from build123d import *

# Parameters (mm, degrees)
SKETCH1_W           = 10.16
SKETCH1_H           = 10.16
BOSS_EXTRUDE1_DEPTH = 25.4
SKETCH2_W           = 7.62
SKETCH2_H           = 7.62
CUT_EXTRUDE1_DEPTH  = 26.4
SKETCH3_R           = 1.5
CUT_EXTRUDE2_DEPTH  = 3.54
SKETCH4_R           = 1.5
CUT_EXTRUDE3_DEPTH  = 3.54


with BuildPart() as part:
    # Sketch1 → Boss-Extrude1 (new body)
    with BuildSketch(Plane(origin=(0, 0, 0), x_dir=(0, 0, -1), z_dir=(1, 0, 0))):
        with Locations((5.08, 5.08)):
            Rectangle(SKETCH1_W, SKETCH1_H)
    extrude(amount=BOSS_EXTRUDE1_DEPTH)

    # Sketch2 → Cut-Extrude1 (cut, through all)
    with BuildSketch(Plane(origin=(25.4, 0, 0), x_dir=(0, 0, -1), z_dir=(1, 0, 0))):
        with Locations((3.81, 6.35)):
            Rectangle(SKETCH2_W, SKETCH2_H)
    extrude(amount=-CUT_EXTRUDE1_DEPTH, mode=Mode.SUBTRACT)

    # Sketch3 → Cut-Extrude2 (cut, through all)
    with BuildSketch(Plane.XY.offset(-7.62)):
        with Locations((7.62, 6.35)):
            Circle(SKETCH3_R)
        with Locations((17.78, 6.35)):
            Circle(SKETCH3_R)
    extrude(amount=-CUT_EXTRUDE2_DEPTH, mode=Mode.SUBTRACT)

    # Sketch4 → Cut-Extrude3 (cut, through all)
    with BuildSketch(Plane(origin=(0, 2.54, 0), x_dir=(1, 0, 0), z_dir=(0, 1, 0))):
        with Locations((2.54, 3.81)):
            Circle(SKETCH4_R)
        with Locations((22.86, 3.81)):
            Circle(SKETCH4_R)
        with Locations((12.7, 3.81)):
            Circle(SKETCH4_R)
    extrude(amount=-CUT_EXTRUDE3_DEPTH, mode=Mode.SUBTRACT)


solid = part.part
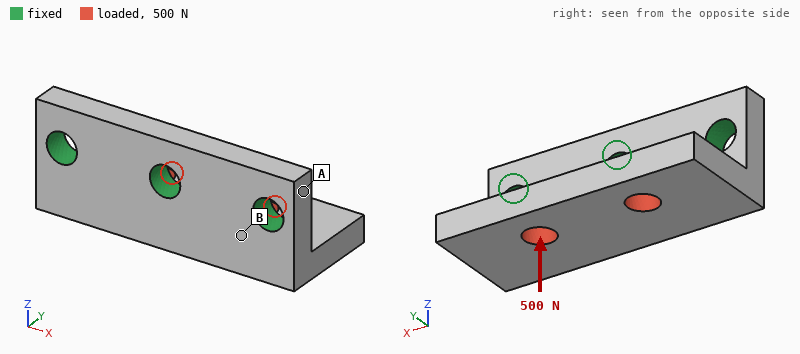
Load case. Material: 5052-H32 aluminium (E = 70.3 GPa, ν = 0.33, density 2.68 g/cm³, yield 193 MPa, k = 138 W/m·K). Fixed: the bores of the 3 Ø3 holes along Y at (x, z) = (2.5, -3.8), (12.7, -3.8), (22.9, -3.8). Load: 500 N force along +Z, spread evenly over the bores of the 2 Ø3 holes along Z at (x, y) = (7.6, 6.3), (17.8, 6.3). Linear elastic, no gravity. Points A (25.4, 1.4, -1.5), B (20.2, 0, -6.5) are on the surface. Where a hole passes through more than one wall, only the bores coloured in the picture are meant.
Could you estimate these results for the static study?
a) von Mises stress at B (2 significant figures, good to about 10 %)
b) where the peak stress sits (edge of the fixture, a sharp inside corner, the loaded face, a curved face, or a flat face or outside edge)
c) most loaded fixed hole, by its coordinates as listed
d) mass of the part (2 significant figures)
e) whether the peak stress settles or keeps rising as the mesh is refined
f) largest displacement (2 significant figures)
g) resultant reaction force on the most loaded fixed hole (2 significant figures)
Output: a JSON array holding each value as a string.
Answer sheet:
["63 MPa", "edge of the fixture", "(12.7, -3.8)", "2.8 g", "keeps rising", "58 µm", "300 N"]
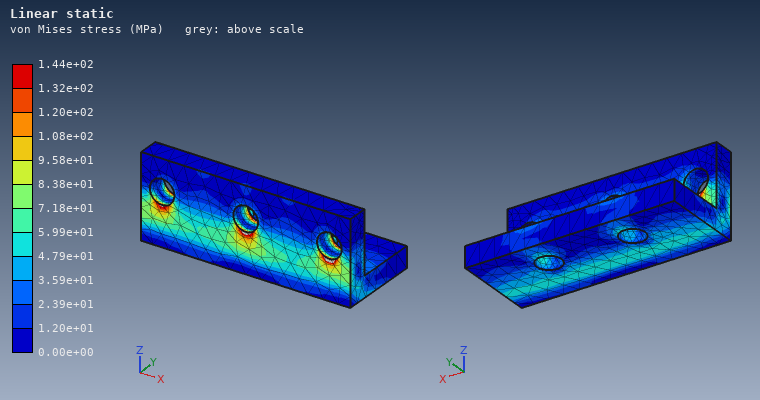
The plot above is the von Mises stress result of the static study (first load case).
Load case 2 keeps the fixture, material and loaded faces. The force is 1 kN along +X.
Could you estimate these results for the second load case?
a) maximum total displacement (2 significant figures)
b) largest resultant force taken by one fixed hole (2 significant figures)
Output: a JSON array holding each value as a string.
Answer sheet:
["22 µm", "440 N"]
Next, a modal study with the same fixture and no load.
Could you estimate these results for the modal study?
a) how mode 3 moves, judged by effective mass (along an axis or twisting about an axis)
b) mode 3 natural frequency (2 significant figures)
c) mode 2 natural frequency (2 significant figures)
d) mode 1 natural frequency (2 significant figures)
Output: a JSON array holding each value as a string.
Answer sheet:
["along X", "41 kHz", "22 kHz", "16 kHz"]
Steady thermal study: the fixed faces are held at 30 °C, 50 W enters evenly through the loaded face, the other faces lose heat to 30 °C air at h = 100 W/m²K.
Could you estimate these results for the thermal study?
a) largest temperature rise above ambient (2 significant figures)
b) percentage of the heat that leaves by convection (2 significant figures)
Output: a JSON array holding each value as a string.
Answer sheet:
["62 K", "5.0 %"]
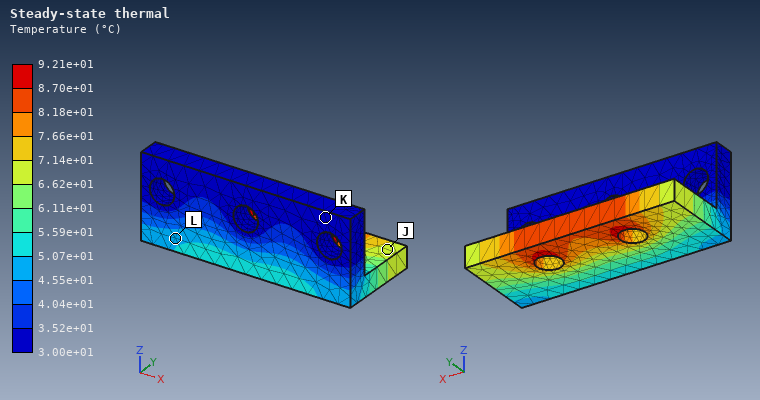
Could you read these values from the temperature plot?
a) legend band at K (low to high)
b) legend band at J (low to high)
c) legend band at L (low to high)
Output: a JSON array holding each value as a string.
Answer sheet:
["3.00e+01 to 3.52e+01 °C", "6.62e+01 to 7.14e+01 °C", "4.55e+01 to 5.07e+01 °C"]
